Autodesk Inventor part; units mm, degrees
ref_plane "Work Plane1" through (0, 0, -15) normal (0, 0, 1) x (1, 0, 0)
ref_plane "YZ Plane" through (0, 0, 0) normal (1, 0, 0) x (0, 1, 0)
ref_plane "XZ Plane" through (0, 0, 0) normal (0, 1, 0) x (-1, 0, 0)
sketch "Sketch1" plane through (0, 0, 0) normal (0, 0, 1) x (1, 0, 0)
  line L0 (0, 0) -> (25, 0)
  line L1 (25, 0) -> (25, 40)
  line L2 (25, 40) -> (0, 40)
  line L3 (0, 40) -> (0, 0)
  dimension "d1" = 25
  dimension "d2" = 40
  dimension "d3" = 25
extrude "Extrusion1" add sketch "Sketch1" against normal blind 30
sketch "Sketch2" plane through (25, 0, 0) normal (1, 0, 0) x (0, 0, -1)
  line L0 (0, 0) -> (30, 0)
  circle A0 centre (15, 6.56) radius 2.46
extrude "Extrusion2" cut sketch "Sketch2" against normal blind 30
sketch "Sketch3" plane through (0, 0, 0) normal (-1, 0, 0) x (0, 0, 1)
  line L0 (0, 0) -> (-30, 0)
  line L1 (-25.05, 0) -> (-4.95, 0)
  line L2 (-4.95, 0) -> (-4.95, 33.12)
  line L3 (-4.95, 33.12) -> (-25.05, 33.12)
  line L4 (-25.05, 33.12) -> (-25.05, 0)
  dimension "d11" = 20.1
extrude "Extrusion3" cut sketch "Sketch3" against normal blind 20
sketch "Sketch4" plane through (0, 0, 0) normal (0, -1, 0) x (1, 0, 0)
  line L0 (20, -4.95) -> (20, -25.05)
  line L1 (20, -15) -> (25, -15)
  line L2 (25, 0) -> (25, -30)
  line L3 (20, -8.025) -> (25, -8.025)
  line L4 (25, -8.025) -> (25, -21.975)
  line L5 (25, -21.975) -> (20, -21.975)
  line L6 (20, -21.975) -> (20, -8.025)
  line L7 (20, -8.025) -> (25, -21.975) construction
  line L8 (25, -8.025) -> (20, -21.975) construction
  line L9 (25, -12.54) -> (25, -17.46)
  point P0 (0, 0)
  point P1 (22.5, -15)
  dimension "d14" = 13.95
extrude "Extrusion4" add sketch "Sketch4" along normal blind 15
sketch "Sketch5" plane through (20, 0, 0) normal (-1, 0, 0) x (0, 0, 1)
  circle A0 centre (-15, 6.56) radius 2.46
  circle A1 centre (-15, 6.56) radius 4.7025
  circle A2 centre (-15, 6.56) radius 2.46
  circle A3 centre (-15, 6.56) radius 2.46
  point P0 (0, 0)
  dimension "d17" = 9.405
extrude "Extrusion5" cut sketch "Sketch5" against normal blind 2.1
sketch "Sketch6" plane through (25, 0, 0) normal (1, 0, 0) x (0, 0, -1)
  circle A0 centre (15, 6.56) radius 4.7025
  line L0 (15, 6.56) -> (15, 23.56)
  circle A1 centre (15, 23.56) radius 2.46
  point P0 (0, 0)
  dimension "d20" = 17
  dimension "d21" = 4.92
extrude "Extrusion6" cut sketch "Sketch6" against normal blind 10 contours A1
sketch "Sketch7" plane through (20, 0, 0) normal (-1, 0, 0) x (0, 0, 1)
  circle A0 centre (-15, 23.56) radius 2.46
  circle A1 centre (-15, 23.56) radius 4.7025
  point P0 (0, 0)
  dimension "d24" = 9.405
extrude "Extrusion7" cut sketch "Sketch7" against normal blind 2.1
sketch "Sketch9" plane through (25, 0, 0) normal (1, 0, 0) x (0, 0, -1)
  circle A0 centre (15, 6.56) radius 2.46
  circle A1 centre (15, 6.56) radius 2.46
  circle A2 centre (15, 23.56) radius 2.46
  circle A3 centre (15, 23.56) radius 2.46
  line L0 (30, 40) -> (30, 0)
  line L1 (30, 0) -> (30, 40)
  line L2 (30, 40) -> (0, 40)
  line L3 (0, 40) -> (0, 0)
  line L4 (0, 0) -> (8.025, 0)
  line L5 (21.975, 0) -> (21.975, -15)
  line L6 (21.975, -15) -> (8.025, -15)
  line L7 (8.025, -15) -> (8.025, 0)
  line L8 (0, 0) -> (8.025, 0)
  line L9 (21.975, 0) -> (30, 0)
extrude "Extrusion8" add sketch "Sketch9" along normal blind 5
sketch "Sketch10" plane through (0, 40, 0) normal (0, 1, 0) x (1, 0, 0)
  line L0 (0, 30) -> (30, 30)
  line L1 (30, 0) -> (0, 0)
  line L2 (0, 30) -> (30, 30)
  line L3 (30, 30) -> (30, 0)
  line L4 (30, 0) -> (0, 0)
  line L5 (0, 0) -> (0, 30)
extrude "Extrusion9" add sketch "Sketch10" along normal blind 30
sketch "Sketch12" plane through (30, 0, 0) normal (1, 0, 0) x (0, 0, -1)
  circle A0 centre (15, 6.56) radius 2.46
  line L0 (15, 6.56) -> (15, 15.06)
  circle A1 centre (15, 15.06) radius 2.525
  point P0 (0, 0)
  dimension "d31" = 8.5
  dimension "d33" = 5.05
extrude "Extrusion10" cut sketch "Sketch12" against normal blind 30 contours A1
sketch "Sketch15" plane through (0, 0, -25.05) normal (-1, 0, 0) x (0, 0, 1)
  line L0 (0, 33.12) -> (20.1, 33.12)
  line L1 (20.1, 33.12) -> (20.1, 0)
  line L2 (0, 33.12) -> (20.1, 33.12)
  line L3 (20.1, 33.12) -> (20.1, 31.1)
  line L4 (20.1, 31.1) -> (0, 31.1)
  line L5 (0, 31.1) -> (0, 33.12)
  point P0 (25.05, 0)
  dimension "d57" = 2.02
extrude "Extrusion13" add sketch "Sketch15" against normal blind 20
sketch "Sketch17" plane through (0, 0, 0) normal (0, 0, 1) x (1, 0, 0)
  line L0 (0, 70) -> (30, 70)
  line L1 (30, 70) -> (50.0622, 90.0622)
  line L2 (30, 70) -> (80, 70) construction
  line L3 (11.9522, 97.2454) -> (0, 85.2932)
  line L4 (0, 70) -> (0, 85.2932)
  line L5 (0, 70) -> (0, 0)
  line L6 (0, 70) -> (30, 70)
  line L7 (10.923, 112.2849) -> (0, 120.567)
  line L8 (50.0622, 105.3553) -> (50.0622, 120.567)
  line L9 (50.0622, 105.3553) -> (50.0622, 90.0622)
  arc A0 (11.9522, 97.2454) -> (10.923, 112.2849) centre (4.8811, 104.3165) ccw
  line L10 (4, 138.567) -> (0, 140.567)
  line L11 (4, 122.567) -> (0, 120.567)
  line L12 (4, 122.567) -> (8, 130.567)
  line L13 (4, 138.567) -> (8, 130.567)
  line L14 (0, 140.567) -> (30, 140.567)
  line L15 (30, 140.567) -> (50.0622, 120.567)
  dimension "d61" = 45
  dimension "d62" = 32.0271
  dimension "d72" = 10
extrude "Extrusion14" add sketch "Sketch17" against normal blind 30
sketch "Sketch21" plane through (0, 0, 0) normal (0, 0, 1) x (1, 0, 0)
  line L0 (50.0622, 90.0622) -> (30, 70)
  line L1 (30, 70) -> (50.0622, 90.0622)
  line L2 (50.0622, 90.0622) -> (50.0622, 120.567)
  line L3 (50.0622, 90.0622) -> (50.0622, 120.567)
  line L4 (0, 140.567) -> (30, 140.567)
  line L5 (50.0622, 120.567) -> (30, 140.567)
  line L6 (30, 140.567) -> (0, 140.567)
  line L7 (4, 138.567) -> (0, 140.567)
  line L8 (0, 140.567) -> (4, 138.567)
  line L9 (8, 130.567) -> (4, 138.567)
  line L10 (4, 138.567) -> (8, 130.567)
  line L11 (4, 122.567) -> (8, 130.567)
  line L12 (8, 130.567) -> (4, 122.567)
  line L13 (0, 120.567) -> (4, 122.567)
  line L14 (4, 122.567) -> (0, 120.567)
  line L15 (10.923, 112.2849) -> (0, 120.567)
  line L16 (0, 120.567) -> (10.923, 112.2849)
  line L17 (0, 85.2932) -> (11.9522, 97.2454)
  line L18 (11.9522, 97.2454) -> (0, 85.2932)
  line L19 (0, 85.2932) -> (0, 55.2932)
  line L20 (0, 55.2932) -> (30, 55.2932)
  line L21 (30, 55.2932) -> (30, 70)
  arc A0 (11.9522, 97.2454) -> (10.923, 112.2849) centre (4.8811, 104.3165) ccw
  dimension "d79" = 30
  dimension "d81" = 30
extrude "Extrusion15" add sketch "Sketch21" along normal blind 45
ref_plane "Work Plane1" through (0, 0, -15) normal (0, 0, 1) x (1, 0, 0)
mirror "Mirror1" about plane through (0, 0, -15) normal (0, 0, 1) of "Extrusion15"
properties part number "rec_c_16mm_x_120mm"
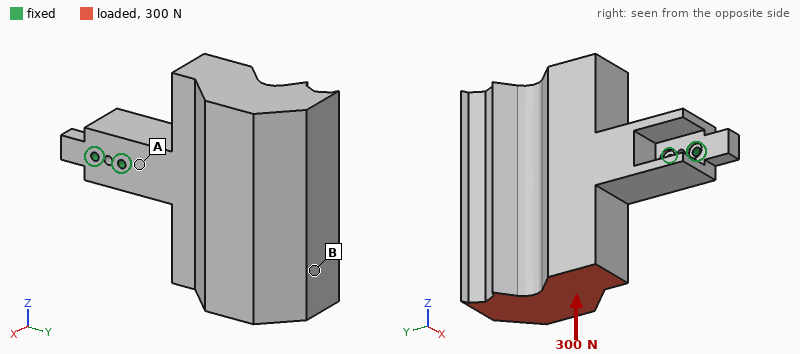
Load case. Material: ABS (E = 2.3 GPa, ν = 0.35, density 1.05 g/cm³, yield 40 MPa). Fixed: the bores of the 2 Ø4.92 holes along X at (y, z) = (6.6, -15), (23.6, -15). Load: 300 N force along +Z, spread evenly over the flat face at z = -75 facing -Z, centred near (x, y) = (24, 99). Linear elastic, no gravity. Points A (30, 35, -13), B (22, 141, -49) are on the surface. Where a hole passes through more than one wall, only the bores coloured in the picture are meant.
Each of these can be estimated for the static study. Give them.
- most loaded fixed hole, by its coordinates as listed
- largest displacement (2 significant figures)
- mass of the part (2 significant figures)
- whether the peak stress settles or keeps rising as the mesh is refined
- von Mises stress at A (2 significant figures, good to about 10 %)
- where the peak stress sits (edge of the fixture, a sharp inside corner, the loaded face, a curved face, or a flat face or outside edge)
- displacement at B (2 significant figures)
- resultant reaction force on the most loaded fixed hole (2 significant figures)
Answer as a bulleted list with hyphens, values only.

- (23.6, -15)
- 1.8 mm
- 440 g
- keeps rising
- 3.7 MPa
- edge of the fixture
- 1.7 mm
- 1.3 kN
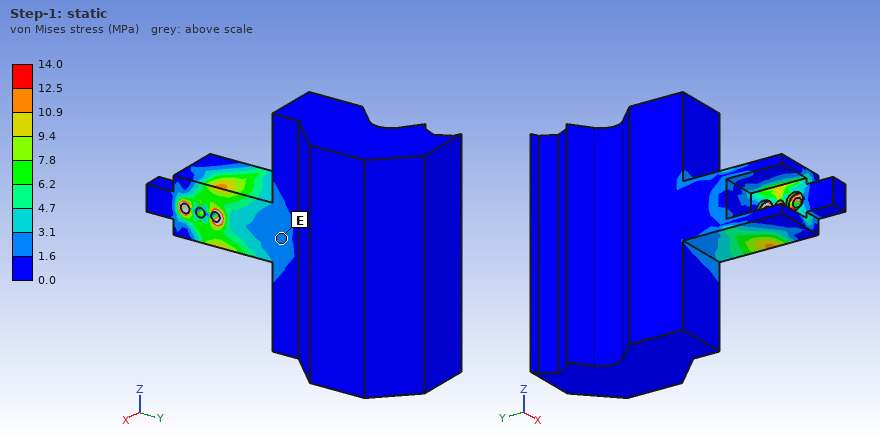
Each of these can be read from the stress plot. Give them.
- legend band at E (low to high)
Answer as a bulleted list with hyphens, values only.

- 1.6 to 3.1 MPa
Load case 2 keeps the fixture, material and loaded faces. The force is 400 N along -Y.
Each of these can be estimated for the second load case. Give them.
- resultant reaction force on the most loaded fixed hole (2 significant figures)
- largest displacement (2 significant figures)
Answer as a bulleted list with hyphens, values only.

- 1.1 kN
- 2.2 mm
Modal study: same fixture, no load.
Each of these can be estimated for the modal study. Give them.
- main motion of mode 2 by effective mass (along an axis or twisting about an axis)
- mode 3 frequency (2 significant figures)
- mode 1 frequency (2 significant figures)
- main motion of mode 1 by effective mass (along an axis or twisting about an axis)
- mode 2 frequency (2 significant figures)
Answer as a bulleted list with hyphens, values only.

- along Z
- 170 Hz
- 110 Hz
- along X
- 120 Hz
